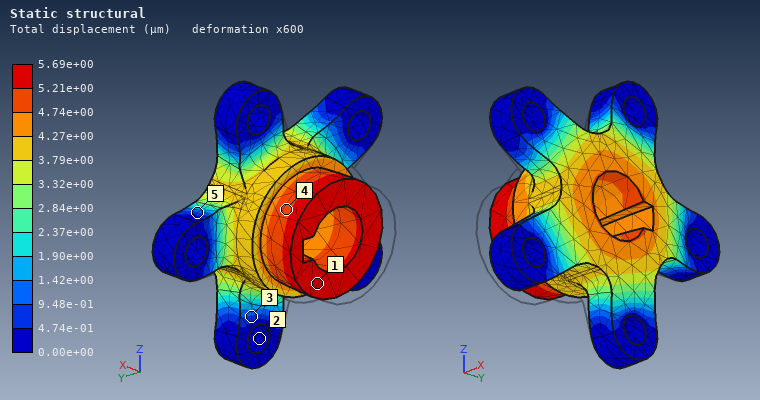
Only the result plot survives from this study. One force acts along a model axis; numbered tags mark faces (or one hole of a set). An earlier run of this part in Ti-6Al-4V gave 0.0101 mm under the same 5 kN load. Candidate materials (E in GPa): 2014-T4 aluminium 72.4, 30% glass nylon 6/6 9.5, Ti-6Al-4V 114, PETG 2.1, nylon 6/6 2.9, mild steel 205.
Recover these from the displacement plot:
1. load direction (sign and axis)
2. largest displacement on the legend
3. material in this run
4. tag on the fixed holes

+X
5.69e+00 µm
mild steel
2
